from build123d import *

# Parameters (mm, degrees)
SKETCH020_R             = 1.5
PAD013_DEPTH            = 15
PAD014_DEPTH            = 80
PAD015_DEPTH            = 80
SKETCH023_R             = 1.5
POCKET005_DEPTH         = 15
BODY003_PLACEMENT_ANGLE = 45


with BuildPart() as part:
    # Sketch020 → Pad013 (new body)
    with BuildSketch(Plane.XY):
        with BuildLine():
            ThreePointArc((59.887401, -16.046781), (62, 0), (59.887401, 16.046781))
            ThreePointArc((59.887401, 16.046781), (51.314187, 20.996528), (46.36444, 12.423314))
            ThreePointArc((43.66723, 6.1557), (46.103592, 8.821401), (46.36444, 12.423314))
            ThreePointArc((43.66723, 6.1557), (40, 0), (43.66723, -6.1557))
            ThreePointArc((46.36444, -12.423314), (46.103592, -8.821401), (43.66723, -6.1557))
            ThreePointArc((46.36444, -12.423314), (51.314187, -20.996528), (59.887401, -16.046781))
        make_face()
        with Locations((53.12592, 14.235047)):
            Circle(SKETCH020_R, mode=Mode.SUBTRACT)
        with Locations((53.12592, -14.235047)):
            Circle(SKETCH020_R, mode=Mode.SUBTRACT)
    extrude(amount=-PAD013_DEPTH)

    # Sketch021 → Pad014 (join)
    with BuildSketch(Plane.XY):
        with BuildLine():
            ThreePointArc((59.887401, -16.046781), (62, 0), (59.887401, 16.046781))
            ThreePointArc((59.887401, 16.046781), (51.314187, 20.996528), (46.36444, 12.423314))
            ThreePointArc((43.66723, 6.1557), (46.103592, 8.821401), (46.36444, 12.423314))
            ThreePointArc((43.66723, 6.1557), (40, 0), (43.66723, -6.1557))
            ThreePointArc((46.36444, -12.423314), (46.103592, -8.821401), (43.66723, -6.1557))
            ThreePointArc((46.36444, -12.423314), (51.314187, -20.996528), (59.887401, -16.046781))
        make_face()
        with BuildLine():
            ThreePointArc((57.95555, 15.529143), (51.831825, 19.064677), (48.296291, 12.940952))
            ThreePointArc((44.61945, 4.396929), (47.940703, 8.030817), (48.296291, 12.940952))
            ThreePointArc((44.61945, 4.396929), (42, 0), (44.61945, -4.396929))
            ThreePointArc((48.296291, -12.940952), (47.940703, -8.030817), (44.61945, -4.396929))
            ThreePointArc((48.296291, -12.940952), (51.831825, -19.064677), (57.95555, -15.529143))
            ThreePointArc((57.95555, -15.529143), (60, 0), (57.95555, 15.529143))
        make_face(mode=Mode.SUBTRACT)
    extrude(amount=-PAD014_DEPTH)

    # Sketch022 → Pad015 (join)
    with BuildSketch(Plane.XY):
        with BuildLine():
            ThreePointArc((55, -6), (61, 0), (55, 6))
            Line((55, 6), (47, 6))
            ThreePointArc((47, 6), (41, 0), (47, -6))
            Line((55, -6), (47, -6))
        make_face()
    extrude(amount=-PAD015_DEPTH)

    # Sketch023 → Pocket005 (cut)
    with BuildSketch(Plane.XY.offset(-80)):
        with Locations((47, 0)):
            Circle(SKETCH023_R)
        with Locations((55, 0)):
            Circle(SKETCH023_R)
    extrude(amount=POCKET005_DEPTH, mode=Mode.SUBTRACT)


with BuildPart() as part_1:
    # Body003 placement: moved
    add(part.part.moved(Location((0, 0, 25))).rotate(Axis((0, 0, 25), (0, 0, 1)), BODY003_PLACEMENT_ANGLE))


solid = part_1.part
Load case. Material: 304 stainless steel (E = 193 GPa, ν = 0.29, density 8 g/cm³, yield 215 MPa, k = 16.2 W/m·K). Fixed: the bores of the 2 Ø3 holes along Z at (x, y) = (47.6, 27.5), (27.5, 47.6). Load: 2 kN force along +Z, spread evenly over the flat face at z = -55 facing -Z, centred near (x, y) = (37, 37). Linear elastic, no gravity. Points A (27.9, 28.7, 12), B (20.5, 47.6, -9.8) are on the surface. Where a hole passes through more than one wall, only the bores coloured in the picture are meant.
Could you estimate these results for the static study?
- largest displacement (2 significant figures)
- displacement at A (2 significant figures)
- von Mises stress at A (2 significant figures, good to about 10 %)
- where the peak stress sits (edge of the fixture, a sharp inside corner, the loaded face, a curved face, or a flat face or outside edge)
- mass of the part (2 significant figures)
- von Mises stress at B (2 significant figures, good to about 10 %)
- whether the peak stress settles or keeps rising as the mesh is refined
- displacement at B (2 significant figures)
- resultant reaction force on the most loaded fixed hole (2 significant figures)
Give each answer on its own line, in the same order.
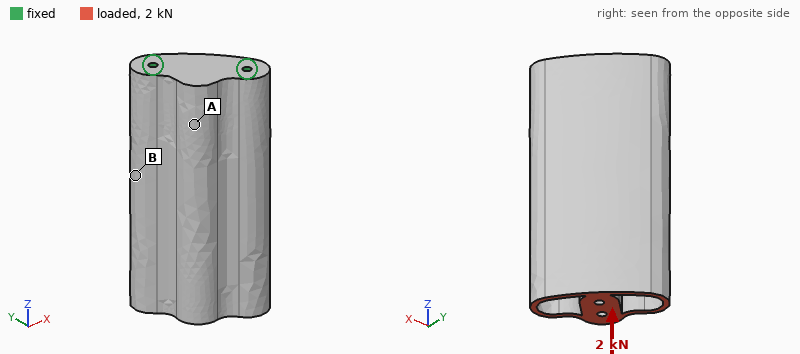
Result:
3.1 µm
0.98 µm
2.1 MPa
edge of the fixture
280 g
6.1 MPa
keeps rising
1.2 µm
1.0 kN
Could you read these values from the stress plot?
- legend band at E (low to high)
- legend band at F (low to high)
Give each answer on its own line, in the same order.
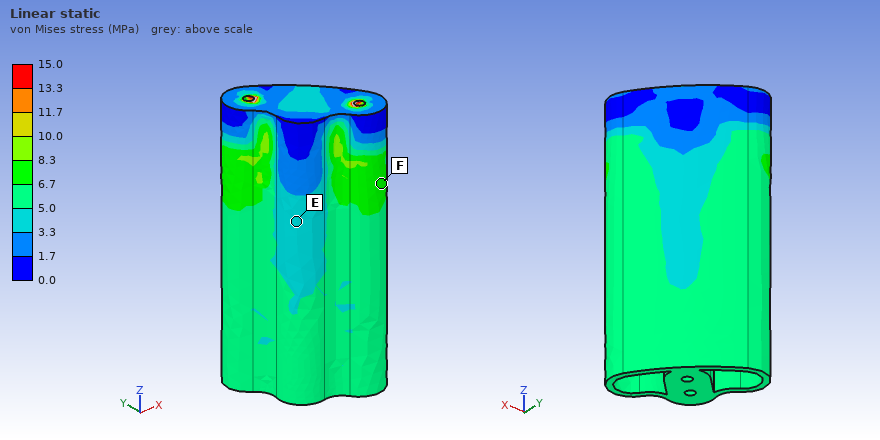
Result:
3.3 to 5.0 MPa
6.7 to 8.3 MPa
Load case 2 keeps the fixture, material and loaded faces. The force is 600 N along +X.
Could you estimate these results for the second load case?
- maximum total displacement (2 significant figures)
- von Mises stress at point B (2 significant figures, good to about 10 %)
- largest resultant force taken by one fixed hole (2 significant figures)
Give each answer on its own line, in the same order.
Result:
38 µm
17 MPa
970 N
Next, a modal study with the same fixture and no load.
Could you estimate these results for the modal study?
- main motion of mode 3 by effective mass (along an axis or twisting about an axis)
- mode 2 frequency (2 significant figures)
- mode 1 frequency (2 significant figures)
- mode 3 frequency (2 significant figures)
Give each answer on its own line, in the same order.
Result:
twisting about Z
4300 Hz
2200 Hz
8200 Hz
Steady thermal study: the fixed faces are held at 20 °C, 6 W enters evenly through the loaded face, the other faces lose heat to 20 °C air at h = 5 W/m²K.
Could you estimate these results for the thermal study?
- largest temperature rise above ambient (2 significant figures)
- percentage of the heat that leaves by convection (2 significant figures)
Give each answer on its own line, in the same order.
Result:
55 K
33 %
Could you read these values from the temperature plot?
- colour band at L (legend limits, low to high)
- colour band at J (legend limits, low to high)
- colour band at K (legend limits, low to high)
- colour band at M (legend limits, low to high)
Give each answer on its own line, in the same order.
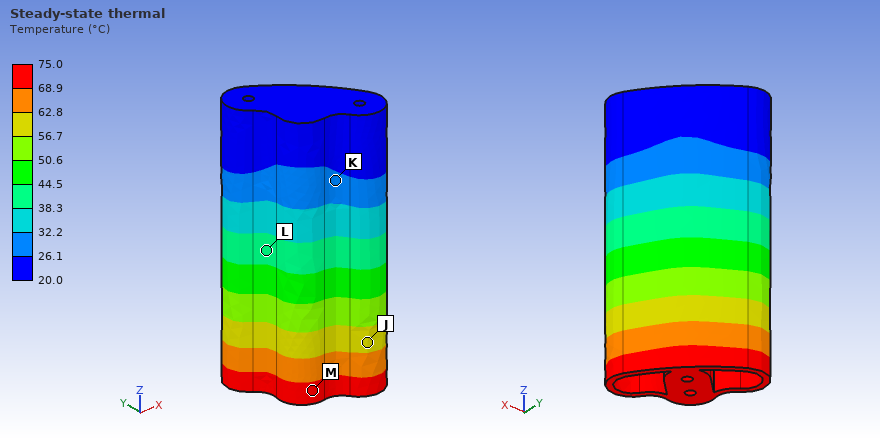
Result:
38.3 to 44.5 °C
56.7 to 62.8 °C
26.1 to 32.2 °C
68.9 to 75.0 °C
